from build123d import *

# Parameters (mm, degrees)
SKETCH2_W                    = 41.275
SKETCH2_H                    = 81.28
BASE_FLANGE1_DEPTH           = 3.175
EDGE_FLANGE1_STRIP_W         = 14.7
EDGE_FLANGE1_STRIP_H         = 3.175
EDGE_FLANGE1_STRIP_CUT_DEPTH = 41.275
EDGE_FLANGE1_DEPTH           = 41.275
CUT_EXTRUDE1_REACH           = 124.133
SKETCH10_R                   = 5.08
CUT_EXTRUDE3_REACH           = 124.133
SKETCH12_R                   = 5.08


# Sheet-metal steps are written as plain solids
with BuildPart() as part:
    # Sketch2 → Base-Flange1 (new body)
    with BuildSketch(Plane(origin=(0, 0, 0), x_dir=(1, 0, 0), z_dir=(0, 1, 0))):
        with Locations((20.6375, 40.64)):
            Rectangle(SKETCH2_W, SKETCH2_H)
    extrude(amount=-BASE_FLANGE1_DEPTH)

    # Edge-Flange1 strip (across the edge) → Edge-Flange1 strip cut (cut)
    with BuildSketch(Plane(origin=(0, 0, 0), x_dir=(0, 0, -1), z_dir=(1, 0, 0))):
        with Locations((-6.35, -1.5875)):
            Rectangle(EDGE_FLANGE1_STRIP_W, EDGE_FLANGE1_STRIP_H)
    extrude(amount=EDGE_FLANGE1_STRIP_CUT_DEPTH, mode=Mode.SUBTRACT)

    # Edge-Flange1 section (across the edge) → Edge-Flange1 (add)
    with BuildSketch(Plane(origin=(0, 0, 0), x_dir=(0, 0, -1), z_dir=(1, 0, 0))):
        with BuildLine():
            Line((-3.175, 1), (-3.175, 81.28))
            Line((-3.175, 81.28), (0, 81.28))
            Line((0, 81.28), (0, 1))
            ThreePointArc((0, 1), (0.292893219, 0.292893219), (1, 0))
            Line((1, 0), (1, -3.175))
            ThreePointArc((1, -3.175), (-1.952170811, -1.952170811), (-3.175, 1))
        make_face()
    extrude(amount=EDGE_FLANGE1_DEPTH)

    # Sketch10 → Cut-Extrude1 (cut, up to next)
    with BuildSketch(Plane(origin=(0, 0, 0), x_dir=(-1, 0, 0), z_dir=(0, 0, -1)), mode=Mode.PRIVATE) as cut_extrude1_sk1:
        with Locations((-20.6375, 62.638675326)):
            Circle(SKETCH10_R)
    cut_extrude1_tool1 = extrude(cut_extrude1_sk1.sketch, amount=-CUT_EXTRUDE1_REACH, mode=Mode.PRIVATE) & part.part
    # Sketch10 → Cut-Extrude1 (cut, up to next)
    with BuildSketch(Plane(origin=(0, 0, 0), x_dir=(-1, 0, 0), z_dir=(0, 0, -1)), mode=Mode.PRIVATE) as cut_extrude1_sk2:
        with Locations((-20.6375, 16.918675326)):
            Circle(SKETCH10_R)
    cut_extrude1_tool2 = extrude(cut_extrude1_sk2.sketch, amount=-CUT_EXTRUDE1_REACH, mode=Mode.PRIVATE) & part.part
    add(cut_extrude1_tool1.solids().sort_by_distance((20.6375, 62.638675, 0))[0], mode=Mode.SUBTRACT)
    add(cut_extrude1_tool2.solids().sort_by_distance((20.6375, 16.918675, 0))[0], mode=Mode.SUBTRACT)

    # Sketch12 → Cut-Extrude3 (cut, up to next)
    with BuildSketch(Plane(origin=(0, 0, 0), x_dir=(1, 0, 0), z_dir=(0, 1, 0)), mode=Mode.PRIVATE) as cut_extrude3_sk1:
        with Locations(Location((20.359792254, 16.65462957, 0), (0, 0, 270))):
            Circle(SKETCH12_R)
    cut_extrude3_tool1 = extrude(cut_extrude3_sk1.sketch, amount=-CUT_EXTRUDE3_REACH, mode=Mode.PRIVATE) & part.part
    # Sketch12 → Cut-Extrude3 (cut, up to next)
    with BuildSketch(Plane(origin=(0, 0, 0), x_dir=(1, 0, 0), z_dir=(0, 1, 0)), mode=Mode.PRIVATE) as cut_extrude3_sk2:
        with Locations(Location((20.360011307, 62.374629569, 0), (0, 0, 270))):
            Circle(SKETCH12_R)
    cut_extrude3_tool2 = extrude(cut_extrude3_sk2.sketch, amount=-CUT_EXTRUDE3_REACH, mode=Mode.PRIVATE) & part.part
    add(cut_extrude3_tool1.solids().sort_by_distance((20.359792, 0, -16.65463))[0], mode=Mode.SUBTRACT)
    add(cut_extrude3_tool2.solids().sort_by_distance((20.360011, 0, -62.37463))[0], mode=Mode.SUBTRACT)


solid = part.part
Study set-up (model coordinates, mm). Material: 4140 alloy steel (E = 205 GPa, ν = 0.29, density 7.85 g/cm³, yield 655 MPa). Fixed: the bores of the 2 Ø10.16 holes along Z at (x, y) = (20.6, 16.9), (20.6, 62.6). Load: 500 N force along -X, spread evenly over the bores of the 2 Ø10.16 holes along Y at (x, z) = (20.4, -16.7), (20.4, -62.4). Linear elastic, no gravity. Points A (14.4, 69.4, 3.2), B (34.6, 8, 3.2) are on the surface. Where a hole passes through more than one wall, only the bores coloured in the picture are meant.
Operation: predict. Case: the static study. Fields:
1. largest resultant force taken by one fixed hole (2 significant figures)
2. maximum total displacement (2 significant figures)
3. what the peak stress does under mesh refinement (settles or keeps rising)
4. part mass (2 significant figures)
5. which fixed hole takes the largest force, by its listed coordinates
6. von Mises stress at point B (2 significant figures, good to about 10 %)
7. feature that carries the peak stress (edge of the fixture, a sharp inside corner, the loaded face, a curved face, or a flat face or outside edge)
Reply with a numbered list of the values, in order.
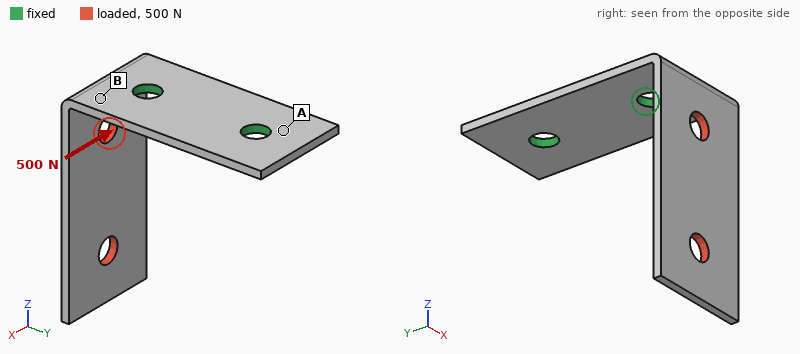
1. 610 N
2. 0.58 mm
3. keeps rising
4. 160 g
5. (20.6, 16.9)
6. 88 MPa
7. edge of the fixture
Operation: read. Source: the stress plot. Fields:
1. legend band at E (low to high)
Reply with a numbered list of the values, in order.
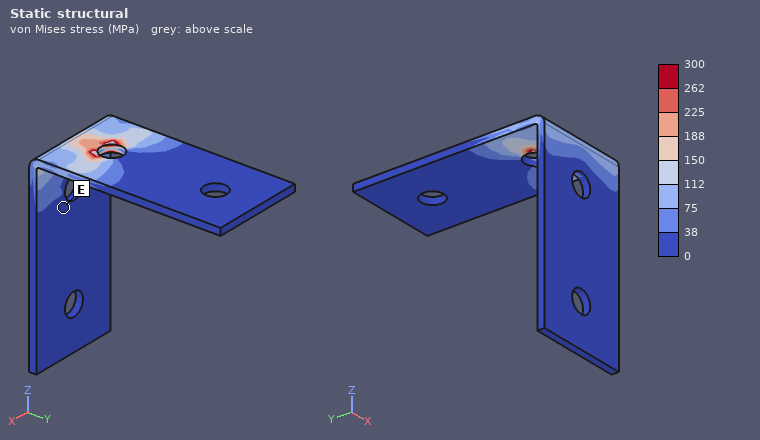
1. 0 to 38 MPa
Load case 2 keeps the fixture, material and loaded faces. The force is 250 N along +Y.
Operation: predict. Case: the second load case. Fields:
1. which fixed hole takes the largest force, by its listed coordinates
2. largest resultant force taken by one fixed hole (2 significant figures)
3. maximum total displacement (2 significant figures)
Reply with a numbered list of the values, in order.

1. (20.6, 16.9)
2. 230 N
3. 1.4 mm
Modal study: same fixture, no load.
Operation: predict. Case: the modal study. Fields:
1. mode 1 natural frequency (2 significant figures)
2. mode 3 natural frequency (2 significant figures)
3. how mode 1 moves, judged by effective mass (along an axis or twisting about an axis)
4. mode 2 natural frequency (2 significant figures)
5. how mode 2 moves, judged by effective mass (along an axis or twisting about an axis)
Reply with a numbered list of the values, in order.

1. 290 Hz
2. 1500 Hz
3. along Y
4. 620 Hz
5. along X
